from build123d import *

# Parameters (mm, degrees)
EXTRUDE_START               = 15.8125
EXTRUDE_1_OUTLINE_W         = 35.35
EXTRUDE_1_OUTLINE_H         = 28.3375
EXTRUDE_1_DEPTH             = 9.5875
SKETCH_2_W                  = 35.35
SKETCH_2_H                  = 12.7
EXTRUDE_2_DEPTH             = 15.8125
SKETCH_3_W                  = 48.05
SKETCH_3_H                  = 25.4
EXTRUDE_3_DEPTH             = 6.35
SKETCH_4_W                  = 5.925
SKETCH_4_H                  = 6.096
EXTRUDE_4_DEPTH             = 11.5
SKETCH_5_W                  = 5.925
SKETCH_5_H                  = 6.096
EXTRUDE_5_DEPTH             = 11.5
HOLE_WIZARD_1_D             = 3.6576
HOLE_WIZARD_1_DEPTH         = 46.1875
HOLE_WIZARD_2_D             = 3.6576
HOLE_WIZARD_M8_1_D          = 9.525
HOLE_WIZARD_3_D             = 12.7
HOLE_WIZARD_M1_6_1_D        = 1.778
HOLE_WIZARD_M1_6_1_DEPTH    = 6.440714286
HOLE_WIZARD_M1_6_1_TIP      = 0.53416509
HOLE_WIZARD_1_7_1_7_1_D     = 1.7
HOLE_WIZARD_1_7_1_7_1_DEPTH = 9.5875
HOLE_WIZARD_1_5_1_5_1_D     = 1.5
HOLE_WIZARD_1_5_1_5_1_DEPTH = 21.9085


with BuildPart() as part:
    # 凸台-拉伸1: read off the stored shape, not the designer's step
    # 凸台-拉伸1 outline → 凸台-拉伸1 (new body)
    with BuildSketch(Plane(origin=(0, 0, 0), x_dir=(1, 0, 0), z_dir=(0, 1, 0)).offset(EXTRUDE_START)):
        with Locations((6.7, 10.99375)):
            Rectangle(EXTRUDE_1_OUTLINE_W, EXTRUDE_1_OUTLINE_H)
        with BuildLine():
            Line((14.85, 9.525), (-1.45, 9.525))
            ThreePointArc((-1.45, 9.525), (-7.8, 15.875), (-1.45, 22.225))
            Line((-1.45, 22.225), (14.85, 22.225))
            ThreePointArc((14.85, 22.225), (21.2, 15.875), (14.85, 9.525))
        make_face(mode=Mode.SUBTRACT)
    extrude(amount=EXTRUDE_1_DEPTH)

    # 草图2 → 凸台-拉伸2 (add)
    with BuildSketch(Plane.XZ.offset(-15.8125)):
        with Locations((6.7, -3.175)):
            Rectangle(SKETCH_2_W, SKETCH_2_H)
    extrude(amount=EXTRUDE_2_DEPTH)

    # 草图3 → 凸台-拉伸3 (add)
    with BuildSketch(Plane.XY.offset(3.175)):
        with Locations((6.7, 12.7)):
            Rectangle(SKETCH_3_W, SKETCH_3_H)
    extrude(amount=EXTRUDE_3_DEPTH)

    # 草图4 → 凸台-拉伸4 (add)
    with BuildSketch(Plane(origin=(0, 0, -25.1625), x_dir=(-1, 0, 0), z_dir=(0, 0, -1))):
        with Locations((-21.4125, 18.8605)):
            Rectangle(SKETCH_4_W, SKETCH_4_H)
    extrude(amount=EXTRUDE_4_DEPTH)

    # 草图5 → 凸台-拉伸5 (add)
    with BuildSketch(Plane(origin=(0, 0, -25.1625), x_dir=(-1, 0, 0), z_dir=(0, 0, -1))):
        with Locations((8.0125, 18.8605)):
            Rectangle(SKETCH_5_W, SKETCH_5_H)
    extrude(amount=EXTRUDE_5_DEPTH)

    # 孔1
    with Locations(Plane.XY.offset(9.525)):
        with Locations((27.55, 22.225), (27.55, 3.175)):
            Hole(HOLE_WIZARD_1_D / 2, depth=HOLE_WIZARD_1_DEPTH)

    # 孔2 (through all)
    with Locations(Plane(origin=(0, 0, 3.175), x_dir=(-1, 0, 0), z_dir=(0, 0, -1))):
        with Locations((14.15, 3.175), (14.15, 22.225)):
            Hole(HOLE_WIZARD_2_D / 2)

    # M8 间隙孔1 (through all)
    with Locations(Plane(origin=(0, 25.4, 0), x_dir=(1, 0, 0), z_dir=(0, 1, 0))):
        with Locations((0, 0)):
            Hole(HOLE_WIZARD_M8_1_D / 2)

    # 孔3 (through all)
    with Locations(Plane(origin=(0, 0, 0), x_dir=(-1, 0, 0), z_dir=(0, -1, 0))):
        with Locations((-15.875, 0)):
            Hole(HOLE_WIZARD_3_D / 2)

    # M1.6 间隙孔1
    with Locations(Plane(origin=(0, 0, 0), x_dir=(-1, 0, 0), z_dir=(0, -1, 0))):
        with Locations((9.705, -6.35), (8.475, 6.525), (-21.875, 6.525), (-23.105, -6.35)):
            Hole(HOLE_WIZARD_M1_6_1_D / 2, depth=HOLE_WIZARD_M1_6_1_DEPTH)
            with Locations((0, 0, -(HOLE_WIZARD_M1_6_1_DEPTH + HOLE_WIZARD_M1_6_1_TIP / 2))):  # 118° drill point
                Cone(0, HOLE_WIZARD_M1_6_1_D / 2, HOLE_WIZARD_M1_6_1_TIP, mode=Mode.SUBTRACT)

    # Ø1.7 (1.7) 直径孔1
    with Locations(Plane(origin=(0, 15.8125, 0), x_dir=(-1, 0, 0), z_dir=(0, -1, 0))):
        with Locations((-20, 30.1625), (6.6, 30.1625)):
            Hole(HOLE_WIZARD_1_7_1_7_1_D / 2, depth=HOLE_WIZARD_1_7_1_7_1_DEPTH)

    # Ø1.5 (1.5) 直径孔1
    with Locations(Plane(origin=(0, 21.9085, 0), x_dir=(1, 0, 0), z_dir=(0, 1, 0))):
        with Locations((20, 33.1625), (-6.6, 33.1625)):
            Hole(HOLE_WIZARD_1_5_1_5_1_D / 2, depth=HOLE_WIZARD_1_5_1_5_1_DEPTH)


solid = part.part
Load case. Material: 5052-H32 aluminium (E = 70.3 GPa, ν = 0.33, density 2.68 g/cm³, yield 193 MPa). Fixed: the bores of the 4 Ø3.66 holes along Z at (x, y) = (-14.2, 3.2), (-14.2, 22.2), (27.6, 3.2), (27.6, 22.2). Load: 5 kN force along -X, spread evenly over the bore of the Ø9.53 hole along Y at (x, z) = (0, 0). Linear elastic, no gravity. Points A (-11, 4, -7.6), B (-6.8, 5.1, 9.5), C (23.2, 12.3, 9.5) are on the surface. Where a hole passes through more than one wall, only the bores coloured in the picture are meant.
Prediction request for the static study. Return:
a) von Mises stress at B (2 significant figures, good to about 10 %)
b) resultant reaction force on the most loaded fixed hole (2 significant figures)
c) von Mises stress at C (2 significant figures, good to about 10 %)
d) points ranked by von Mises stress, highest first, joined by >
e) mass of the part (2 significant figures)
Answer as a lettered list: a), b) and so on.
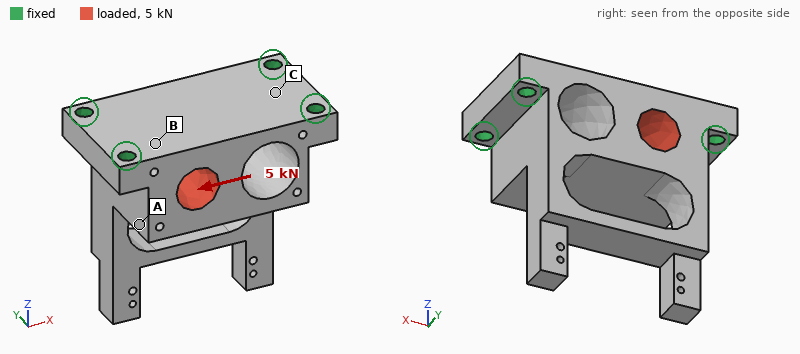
a) 20 MPa
b) 1.9 kN
c) 11 MPa
d) B > C > A
e) 45 g
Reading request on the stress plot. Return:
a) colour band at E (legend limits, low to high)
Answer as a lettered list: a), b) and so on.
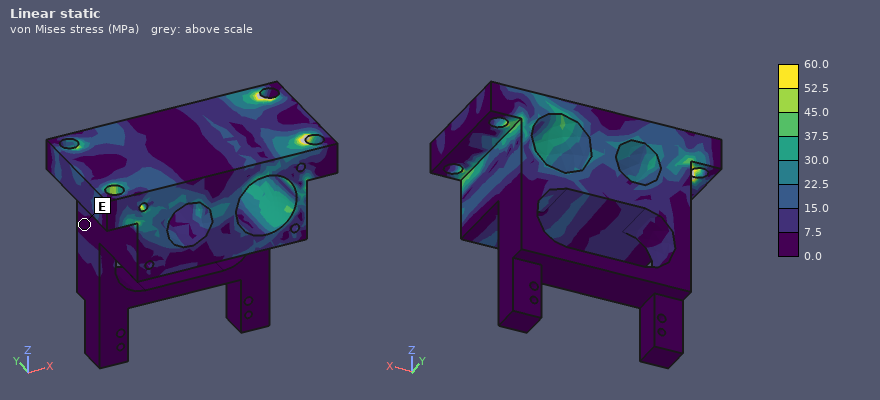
a) 0.0 to 7.5 MPa
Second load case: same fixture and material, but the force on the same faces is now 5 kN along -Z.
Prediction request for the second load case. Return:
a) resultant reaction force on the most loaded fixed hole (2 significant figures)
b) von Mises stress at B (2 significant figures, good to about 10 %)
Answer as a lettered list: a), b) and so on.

a) 1.8 kN
b) 9.6 MPa
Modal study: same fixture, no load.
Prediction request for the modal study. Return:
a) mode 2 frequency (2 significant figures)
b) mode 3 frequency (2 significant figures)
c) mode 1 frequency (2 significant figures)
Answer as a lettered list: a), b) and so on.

a) 6100 Hz
b) 8300 Hz
c) 6100 Hz
